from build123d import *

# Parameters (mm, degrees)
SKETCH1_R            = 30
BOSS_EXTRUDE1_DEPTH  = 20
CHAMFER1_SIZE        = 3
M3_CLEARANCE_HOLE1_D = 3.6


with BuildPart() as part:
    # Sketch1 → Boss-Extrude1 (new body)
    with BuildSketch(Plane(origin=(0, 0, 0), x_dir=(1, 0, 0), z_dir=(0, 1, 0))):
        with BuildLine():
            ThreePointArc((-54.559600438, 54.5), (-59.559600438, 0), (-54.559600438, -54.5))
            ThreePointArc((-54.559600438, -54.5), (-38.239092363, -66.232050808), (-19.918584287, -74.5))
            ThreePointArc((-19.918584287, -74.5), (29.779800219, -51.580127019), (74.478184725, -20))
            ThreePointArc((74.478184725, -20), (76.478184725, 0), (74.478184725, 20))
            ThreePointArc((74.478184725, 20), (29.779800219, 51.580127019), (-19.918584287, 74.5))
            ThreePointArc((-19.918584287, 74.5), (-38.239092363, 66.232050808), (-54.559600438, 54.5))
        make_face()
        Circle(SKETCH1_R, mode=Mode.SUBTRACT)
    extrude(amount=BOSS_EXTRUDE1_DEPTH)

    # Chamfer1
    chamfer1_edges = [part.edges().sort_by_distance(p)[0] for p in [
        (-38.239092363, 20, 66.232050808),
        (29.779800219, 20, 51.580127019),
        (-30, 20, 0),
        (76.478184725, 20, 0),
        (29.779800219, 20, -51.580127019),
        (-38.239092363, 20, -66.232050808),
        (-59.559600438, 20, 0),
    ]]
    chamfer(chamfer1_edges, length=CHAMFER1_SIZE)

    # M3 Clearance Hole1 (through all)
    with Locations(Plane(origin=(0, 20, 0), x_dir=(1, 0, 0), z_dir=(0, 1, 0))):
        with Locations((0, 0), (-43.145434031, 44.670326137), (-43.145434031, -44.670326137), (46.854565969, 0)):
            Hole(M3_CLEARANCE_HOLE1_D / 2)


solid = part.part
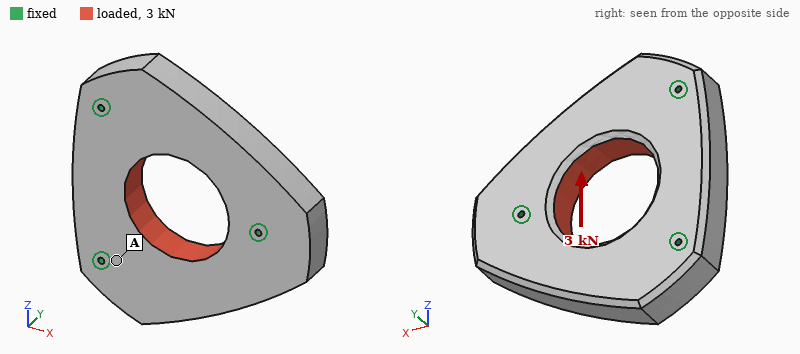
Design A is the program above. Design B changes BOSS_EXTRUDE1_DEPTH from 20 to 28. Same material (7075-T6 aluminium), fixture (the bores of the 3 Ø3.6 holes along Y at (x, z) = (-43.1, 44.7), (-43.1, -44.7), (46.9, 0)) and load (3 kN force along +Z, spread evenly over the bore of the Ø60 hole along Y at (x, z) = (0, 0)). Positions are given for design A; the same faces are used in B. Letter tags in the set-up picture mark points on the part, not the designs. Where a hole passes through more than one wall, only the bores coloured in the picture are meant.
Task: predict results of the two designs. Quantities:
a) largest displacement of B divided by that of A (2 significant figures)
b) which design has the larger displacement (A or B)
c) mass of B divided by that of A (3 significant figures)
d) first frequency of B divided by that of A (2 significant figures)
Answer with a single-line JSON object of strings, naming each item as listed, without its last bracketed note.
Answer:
{"largest displacement of B divided by that of A": "0.69", "which design has the larger displacement": "A", "mass of B divided by that of A": "1.40", "first frequency of B divided by that of A": "1.3"}
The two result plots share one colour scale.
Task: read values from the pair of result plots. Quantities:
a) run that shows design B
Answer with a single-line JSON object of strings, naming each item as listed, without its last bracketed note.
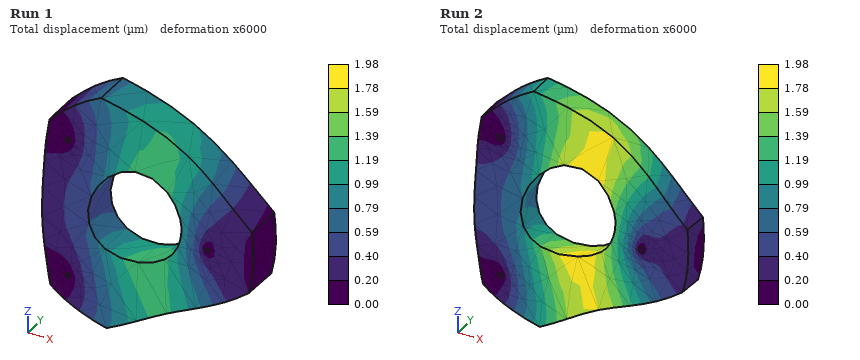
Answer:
{"run that shows design B": "Run 1"}
